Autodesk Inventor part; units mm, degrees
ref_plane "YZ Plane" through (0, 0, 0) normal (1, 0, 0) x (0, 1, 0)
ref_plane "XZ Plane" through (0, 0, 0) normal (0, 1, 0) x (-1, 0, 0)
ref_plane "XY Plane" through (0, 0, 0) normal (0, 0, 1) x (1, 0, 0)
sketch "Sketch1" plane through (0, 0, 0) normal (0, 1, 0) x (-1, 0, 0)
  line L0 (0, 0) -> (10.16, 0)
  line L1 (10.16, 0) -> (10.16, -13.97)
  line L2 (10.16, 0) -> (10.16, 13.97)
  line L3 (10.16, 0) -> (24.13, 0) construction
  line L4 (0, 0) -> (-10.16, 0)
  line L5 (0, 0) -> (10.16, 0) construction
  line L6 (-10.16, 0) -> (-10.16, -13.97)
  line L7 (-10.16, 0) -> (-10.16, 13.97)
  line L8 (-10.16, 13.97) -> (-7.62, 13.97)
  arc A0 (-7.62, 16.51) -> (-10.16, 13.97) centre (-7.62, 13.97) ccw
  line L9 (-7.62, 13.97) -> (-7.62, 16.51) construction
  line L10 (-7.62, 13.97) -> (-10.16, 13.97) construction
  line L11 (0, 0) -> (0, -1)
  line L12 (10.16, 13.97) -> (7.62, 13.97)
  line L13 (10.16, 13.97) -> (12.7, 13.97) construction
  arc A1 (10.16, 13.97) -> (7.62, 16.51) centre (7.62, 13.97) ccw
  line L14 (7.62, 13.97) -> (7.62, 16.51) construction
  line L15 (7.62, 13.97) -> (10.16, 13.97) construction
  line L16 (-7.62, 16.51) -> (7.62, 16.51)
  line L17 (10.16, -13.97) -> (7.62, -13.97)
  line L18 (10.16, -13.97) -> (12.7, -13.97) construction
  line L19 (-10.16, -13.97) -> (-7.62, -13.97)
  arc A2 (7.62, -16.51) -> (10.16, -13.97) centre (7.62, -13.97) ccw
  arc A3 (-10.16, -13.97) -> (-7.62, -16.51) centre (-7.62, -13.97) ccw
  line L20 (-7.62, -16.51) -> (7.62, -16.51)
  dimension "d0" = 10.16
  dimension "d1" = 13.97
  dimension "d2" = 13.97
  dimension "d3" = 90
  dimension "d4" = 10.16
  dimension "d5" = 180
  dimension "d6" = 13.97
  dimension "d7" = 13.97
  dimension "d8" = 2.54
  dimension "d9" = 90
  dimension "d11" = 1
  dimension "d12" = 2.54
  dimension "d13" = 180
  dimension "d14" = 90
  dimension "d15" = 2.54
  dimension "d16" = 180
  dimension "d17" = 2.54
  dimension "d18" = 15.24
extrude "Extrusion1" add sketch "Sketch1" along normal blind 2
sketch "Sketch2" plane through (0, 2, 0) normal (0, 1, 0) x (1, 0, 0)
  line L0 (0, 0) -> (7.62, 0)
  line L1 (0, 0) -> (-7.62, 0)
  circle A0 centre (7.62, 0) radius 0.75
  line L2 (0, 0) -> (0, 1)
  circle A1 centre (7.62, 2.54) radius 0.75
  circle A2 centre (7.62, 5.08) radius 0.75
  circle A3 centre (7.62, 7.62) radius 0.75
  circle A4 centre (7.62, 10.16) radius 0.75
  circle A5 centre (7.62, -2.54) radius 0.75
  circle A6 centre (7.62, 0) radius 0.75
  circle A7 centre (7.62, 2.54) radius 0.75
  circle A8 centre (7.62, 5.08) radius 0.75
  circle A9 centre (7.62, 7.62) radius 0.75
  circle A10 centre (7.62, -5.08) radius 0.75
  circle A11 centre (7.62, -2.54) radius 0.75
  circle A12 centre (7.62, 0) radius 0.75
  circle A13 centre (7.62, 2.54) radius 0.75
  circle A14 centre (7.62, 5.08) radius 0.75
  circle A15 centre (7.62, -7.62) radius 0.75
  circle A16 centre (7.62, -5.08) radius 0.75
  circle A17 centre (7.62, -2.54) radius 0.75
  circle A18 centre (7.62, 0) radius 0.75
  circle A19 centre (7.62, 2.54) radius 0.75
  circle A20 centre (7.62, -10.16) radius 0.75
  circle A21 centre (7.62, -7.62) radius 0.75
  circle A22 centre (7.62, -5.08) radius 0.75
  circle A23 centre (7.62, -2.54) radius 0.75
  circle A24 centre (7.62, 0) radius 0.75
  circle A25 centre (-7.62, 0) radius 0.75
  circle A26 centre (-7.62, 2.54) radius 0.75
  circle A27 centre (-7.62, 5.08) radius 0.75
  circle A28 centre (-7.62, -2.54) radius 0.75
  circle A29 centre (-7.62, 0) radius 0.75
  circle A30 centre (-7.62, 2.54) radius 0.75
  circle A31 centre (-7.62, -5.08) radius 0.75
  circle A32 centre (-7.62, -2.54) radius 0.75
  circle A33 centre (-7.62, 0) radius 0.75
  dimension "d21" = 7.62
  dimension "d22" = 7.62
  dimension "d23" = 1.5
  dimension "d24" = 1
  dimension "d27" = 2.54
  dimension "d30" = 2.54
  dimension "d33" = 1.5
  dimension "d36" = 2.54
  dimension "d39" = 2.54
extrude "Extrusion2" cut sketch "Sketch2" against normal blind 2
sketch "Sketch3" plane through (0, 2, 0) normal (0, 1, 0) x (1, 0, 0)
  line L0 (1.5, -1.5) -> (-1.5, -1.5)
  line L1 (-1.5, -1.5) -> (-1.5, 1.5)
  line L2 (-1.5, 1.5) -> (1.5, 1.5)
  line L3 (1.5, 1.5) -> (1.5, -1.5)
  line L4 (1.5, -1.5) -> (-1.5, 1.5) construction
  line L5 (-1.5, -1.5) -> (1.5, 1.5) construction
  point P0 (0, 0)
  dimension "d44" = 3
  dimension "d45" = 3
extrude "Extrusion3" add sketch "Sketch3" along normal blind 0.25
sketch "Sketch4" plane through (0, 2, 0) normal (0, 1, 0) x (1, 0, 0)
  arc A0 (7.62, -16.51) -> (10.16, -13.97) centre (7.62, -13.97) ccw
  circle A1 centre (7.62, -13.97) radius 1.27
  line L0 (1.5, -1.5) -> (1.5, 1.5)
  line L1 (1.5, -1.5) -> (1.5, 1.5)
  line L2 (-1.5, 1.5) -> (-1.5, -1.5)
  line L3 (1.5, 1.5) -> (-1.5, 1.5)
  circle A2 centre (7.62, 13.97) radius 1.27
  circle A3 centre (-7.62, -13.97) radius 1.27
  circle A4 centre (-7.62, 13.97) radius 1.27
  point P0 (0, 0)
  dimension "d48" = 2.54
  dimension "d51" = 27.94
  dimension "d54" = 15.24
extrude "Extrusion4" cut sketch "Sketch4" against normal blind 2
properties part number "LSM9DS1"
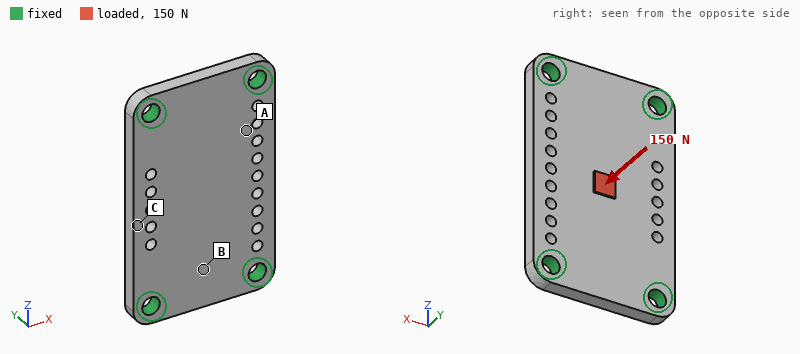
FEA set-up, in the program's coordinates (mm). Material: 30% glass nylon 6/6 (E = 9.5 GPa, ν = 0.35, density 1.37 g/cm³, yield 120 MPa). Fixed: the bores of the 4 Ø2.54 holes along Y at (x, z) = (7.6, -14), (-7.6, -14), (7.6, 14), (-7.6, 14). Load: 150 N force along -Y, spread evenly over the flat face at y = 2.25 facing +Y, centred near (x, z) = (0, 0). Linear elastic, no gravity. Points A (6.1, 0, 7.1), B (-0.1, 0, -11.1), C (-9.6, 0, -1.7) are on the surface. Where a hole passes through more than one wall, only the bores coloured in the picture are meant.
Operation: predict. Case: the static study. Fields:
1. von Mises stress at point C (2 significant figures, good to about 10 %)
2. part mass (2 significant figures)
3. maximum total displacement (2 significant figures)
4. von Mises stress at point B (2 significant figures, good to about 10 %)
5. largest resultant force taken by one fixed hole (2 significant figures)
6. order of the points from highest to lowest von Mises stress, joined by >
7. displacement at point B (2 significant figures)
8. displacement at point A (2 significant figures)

25 MPa
1.7 g
0.17 mm
14 MPa
38 N
C > B > A
0.036 mm
0.072 mm
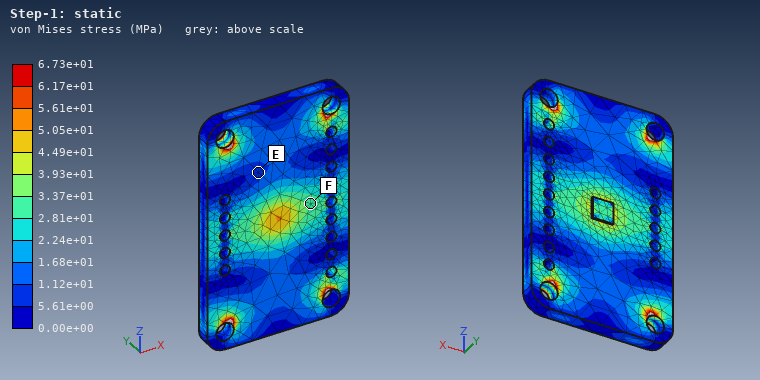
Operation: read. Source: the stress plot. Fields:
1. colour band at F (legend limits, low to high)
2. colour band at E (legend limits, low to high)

2.81e+01 to 3.37e+01 MPa
5.61e+00 to 1.12e+01 MPa
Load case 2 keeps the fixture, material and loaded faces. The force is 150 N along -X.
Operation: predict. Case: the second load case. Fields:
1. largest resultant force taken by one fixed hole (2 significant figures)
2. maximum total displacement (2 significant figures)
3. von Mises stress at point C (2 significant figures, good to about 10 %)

53 N
26 µm
8.5 MPa
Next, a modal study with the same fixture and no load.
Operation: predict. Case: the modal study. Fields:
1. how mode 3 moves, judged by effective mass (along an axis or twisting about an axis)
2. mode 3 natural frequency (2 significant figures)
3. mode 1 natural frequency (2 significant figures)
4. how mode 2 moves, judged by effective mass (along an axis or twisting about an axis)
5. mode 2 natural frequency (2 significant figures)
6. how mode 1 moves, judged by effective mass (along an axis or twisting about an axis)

twisting about X
17 kHz
6700 Hz
twisting about Z
9700 Hz
along Y
